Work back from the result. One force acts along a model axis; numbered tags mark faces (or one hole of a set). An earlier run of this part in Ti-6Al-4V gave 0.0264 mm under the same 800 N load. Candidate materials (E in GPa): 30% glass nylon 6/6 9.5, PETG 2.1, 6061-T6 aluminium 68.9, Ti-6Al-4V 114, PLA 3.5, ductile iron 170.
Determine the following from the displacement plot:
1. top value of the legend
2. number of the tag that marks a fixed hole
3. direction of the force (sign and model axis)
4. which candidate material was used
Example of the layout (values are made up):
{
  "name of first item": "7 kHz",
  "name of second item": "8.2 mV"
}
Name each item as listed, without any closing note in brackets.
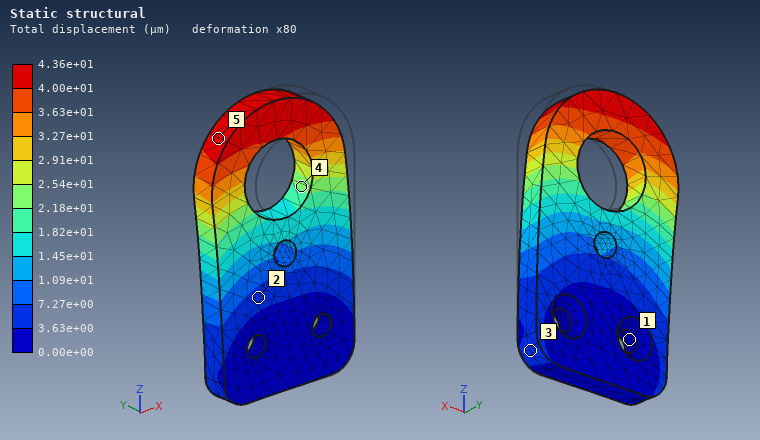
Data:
{
  "top value of the legend": "4.36e+01 µm",
  "number of the tag that marks a fixed hole": "1",
  "direction of the force": "-X",
  "which candidate material was used": "6061-T6 aluminium"
}
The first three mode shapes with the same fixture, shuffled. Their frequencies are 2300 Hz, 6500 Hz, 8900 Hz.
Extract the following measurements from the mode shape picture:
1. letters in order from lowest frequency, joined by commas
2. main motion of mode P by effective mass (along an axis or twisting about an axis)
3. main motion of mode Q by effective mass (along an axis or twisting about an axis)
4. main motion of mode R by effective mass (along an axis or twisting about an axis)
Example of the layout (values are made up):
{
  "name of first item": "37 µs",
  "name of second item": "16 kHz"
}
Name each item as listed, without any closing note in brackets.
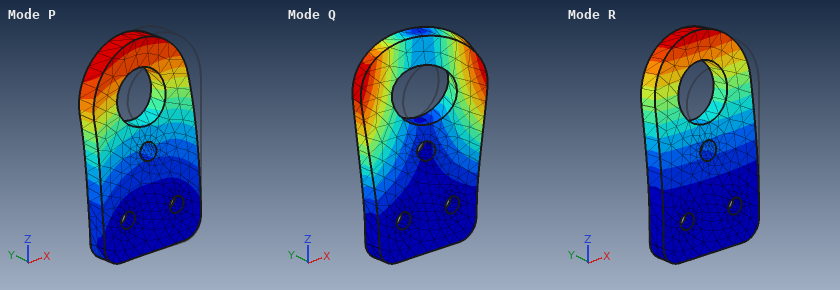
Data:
{
  "letters in order from lowest frequency, joined by commas": "R, Q, P",
  "main motion of mode P by effective mass": "along X",
  "main motion of mode Q by effective mass": "twisting about Z",
  "main motion of mode R by effective mass": "along Y"
}
